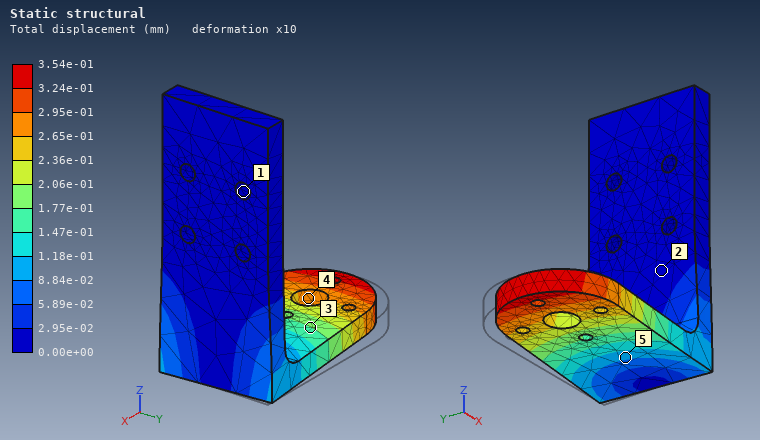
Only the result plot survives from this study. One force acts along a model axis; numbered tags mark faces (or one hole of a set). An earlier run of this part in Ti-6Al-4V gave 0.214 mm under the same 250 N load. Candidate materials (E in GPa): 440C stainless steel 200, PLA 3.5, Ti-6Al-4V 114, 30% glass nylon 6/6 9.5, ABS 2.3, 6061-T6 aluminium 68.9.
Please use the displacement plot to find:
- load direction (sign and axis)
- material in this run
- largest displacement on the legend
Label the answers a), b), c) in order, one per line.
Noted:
a) -Y
b) 6061-T6 aluminium
c) 3.54e-01 mm
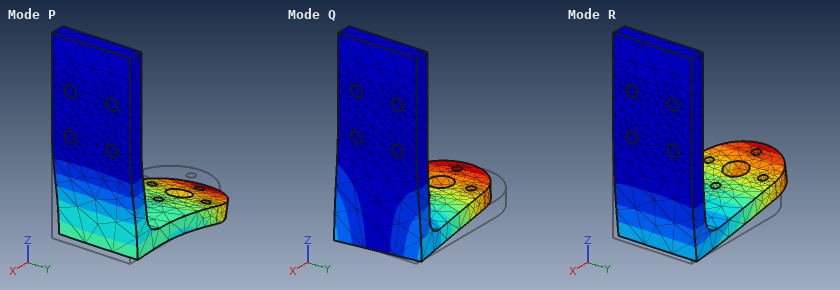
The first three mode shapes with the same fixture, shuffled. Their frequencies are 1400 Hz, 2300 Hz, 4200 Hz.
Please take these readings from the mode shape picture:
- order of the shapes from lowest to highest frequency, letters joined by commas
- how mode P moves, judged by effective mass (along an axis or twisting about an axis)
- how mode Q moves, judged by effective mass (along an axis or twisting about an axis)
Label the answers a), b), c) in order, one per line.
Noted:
a) R, Q, P
b) along X
c) along Y
